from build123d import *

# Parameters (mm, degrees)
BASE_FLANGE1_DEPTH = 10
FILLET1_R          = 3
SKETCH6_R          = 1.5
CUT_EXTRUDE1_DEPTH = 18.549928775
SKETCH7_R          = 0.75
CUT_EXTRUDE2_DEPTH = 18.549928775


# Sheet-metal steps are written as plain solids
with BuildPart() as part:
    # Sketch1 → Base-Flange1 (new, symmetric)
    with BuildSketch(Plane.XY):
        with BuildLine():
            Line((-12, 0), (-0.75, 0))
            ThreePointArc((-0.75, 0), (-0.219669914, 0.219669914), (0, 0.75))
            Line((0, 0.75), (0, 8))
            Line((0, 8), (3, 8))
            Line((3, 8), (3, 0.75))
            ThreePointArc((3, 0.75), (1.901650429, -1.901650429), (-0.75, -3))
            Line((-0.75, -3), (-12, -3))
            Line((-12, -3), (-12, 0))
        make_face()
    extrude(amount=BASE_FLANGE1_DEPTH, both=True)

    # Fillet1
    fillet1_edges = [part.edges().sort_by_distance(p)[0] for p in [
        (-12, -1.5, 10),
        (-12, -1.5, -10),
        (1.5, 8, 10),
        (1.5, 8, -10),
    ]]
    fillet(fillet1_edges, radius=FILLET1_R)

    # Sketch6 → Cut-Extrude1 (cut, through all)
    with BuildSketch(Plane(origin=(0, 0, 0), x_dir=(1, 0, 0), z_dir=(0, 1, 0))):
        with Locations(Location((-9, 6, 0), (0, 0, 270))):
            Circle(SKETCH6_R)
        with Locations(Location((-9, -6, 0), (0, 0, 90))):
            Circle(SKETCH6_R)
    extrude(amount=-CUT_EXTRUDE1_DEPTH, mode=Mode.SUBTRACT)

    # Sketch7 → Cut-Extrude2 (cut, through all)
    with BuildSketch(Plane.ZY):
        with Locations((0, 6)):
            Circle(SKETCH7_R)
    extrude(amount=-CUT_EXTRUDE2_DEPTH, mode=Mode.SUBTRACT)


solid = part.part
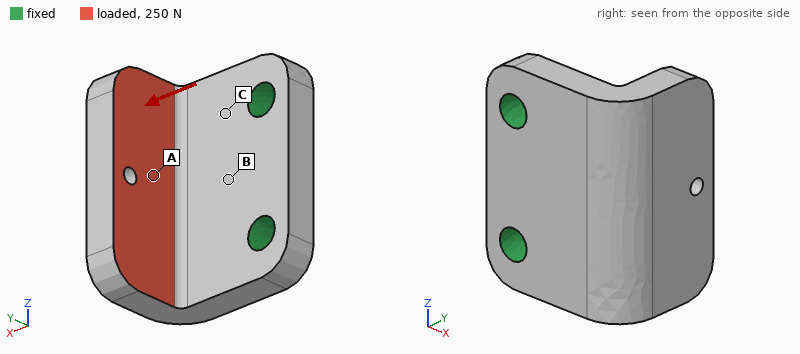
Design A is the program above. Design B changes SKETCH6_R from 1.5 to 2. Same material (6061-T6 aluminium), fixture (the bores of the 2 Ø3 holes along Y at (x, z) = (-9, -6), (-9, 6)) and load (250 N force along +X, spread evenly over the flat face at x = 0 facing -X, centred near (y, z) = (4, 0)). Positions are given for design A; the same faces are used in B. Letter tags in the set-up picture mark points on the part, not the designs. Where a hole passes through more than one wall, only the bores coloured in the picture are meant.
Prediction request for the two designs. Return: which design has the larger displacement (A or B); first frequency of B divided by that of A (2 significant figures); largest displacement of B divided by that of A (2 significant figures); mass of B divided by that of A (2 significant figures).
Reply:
A
1.1
0.92
0.97
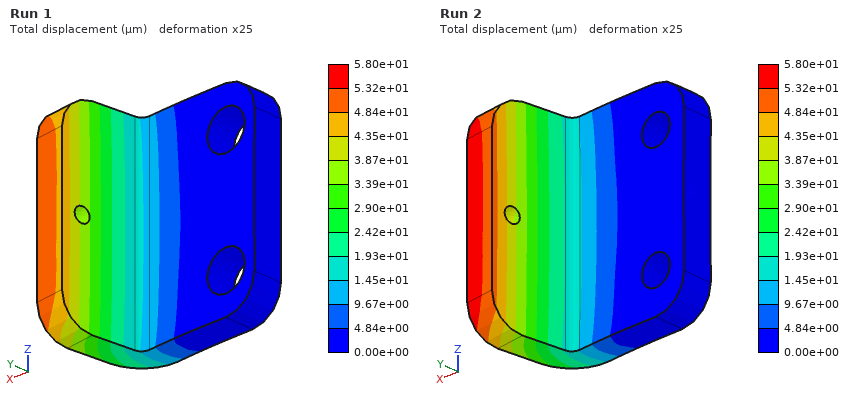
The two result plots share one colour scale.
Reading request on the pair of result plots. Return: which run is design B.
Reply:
Run 1
